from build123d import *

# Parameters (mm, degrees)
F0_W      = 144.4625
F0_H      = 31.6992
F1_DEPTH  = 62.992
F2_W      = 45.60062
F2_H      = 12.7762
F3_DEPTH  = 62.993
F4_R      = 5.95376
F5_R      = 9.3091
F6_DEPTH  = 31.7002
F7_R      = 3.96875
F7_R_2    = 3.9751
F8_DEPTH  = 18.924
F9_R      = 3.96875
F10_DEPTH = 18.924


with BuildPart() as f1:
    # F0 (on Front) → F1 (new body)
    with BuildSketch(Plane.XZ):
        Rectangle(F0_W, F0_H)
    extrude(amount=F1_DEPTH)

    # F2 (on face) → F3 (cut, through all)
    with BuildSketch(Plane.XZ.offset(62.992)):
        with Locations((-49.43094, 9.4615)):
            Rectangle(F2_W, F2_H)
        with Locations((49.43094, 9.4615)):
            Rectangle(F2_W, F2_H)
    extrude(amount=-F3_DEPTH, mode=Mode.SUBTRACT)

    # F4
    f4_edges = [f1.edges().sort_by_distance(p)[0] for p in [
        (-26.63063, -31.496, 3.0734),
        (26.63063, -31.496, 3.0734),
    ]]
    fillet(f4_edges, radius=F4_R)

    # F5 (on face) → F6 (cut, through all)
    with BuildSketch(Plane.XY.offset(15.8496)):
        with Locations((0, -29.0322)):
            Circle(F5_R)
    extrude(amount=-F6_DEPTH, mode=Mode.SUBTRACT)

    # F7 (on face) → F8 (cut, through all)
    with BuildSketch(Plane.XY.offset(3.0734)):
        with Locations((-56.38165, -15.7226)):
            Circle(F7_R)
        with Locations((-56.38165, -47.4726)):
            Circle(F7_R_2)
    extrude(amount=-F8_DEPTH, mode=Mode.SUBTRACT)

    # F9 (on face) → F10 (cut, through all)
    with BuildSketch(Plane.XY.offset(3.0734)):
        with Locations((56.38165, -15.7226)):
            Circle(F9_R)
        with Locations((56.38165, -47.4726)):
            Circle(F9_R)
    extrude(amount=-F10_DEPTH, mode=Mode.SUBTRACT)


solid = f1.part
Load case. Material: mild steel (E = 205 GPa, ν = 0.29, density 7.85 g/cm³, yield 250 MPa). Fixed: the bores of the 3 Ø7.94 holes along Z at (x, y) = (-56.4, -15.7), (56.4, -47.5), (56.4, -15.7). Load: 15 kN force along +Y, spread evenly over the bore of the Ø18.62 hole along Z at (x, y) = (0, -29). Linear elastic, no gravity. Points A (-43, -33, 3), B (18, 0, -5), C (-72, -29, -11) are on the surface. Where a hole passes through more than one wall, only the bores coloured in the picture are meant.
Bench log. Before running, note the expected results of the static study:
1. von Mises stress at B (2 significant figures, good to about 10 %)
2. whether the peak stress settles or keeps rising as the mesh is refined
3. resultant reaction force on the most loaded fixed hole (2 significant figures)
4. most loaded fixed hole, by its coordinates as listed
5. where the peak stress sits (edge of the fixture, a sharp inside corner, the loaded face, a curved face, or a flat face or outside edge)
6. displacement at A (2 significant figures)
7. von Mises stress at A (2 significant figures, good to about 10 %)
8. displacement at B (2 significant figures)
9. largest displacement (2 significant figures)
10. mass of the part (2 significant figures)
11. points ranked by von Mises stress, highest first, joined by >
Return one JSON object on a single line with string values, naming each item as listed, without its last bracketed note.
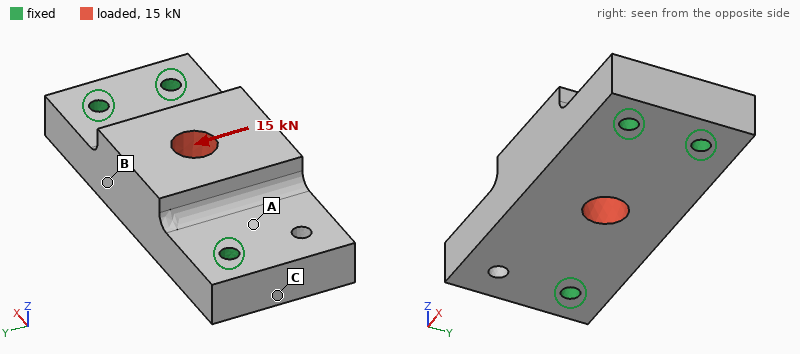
{"von Mises stress at B": "10 MPa", "whether the peak stress settles or keeps rising as the mesh is refined": "keeps rising", "resultant reaction force on the most loaded fixed hole": "7.5 kN", "most loaded fixed hole, by its coordinates as listed": "(56.4, -15.7)", "where the peak stress sits": "edge of the fixture", "displacement at A": "3.9 µm", "von Mises stress at A": "19 MPa", "displacement at B": "6.8 µm", "largest displacement": "12 µm", "mass of the part": "1.6 kg", "points ranked by von Mises stress, highest first, joined by >": "A > B > C"}
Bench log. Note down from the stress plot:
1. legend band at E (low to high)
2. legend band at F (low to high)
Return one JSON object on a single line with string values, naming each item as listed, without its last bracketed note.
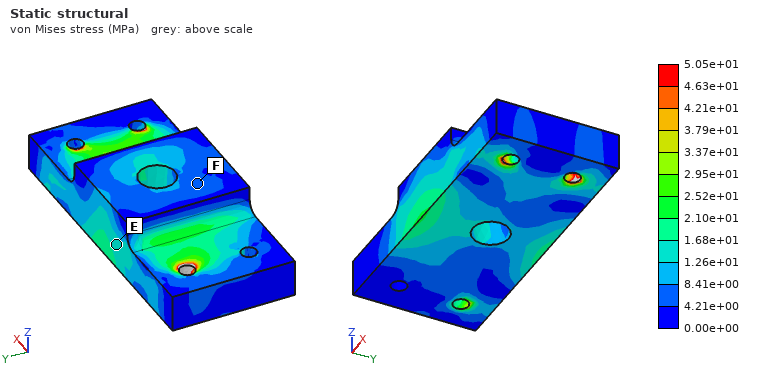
{"legend band at E": "1.26e+01 to 1.68e+01 MPa", "legend band at F": "4.21e+00 to 8.41e+00 MPa"}
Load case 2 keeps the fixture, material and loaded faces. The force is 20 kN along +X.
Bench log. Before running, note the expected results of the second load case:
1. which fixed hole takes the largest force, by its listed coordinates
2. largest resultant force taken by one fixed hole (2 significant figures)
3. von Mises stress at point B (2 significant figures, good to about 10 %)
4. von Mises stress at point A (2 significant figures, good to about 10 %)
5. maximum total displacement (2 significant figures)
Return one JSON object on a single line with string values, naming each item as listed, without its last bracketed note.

{"which fixed hole takes the largest force, by its listed coordinates": "(-56.4, -15.7)", "largest resultant force taken by one fixed hole": "7.8 kN", "von Mises stress at point B": "4.4 MPa", "von Mises stress at point A": "9.4 MPa", "maximum total displacement": "4.5 µm"}
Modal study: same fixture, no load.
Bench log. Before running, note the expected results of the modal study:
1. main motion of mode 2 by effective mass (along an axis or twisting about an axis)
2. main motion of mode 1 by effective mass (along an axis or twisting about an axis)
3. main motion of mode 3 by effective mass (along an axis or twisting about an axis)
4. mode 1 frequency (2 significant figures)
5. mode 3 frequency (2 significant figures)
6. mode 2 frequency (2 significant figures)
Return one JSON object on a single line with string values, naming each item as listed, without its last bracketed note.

{"main motion of mode 2 by effective mass": "along Z", "main motion of mode 1 by effective mass": "along Z", "main motion of mode 3 by effective mass": "along Y", "mode 1 frequency": "4700 Hz", "mode 3 frequency": "8500 Hz", "mode 2 frequency": "6800 Hz"}
